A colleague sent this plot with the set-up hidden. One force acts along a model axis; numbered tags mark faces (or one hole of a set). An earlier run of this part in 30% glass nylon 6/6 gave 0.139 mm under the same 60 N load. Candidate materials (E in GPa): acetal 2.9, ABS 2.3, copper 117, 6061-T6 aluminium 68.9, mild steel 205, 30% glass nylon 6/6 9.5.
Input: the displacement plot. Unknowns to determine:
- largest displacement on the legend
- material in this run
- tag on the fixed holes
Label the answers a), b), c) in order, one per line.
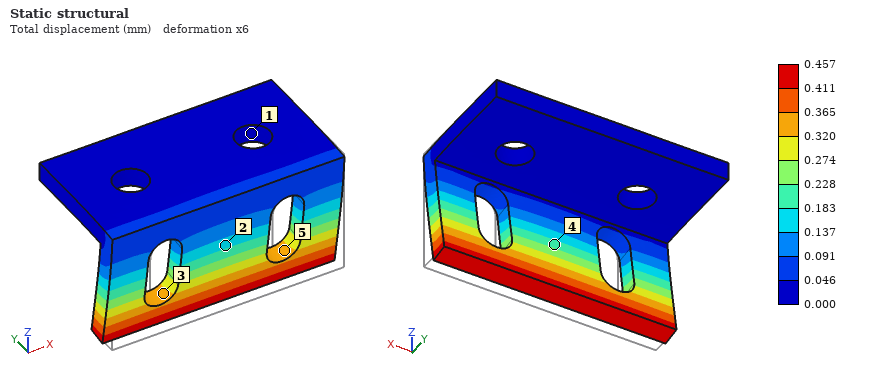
a) 0.457 mm
b) acetal
c) 1
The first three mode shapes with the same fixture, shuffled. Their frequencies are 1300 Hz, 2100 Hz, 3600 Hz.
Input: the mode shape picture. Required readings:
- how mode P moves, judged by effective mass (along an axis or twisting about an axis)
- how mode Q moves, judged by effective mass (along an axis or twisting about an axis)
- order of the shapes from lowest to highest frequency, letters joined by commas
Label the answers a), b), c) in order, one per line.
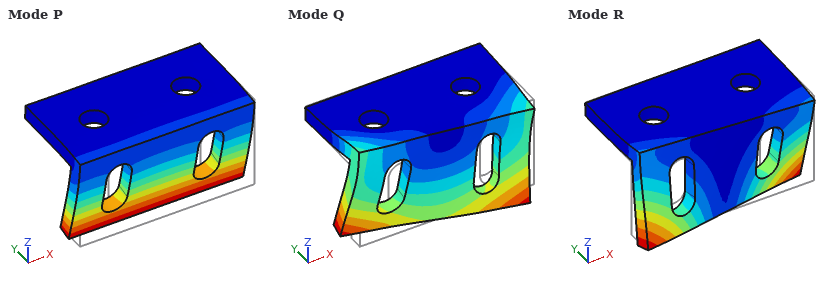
a) along Y
b) along X
c) P, R, Q
